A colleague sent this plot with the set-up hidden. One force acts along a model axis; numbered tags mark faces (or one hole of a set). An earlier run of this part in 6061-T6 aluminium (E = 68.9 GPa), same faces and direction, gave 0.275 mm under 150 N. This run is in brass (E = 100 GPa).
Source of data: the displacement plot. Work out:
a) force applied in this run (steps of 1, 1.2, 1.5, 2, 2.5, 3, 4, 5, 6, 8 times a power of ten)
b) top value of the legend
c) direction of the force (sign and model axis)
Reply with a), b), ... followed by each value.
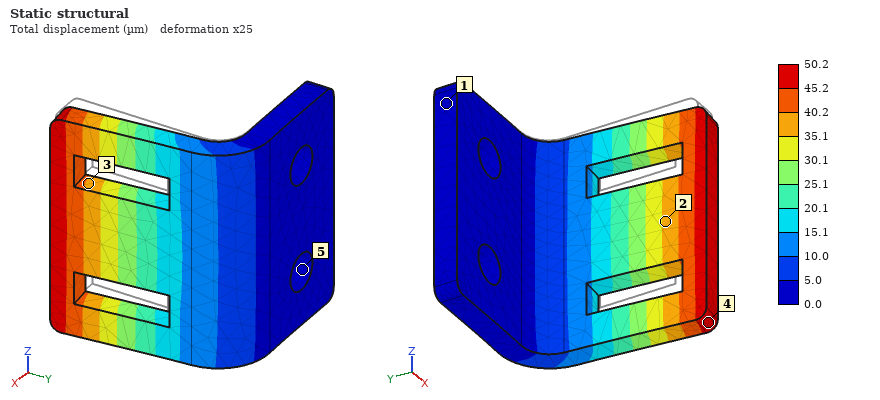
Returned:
a) 40 N
b) 50.2 µm
c) +X
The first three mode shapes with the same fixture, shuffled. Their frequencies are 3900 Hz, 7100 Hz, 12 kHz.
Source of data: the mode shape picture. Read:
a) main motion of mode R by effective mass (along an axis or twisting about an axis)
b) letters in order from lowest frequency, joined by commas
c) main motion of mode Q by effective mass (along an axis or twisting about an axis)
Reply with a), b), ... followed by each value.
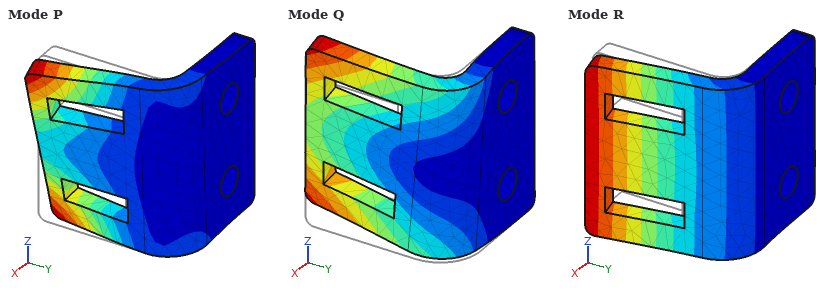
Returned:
a) along X
b) R, Q, P
c) along Z
